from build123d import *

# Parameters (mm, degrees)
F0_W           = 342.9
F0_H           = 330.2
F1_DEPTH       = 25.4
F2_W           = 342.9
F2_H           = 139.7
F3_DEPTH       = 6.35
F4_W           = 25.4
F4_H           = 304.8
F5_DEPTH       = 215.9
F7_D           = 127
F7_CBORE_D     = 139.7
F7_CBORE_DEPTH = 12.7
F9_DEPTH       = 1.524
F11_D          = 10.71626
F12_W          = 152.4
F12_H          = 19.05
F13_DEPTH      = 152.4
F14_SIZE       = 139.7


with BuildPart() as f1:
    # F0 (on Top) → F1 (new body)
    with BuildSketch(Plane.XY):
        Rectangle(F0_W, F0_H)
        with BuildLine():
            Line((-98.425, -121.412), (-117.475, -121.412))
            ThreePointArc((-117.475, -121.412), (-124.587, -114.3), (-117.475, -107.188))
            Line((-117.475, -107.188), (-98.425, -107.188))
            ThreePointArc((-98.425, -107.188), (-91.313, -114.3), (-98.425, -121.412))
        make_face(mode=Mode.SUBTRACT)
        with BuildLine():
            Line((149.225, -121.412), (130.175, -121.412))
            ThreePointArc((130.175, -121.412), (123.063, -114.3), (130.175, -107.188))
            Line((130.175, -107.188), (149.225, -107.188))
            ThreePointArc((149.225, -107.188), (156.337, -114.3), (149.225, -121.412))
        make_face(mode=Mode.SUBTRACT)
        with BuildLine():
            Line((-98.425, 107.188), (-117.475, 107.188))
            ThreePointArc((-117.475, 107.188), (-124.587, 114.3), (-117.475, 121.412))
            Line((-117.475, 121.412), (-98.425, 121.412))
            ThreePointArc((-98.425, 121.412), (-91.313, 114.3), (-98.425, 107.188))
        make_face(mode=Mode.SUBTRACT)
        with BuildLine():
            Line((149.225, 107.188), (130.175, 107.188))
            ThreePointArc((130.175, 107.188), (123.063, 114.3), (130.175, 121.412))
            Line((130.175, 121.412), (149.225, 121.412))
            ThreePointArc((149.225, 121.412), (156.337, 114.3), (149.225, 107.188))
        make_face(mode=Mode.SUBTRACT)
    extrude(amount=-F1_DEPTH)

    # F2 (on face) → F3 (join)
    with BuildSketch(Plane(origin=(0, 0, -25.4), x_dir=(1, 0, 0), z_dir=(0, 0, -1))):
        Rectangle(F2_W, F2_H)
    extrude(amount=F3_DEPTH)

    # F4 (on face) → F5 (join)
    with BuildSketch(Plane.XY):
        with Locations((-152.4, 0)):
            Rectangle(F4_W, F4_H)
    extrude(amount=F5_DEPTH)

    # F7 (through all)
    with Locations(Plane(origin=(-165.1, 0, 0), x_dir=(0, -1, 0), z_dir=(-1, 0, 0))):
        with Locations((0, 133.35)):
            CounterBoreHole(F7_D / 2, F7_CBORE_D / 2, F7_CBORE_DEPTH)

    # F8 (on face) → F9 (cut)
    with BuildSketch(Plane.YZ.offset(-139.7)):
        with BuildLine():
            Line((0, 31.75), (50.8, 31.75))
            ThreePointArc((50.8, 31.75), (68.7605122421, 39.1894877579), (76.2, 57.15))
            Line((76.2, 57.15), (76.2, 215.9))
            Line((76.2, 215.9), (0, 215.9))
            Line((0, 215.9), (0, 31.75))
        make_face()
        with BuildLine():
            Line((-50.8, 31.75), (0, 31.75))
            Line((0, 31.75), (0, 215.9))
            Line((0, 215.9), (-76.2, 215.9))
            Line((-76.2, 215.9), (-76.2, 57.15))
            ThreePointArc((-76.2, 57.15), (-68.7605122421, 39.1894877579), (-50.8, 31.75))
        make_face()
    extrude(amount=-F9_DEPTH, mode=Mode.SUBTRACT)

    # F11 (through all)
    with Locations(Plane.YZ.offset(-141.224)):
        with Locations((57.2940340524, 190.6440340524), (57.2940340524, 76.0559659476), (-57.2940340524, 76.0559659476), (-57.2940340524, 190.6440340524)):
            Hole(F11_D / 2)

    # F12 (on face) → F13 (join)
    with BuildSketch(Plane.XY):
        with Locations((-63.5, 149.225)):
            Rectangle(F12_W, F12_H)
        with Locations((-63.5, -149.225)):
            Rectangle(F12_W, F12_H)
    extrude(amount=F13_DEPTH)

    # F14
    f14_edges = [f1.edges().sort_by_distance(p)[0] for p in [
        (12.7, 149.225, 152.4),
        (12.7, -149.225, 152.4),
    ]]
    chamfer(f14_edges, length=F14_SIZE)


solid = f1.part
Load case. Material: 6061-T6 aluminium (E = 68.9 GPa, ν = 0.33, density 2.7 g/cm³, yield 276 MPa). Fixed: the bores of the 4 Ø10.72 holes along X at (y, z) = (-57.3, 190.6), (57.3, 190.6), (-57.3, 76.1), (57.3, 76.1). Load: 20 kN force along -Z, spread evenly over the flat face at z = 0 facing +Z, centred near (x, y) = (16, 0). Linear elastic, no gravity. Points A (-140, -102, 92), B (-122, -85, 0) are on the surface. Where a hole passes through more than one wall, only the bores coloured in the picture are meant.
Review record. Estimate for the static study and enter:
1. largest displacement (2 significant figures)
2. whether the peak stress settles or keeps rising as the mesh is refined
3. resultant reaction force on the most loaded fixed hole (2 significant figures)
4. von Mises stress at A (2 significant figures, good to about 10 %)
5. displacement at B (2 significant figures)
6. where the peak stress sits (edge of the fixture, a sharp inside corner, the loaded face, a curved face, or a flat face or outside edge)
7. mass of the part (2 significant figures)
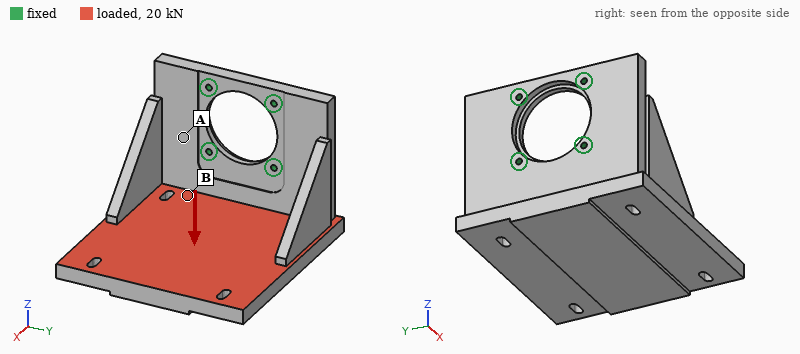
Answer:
2.1 mm
keeps rising
14 kN
52 MPa
0.32 mm
edge of the fixture
13 kg
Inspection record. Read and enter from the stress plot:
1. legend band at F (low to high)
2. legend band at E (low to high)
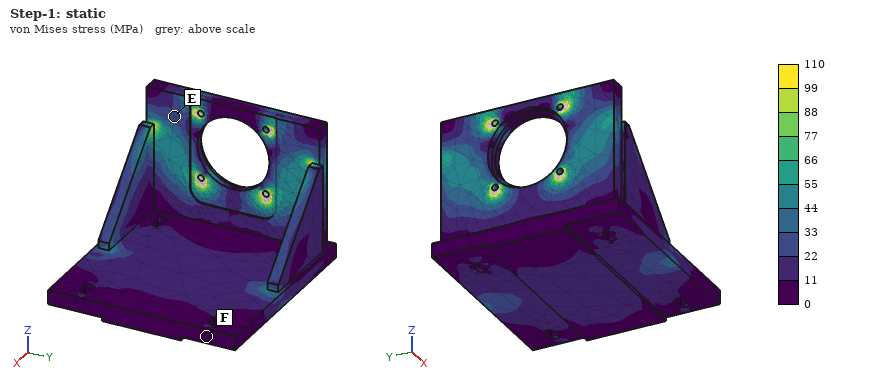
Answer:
0 to 11 MPa
22 to 33 MPa
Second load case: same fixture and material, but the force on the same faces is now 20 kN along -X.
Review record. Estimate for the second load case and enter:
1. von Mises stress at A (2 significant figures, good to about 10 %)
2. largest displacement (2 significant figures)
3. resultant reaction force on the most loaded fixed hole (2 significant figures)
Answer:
20 MPa
0.51 mm
13 kN
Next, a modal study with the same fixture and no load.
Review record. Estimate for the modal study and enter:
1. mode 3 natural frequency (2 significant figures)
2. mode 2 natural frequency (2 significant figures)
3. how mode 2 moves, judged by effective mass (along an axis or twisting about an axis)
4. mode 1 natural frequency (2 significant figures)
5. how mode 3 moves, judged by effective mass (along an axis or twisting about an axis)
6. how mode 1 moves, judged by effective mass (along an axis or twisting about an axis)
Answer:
670 Hz
270 Hz
along Y
210 Hz
along X
along Z
